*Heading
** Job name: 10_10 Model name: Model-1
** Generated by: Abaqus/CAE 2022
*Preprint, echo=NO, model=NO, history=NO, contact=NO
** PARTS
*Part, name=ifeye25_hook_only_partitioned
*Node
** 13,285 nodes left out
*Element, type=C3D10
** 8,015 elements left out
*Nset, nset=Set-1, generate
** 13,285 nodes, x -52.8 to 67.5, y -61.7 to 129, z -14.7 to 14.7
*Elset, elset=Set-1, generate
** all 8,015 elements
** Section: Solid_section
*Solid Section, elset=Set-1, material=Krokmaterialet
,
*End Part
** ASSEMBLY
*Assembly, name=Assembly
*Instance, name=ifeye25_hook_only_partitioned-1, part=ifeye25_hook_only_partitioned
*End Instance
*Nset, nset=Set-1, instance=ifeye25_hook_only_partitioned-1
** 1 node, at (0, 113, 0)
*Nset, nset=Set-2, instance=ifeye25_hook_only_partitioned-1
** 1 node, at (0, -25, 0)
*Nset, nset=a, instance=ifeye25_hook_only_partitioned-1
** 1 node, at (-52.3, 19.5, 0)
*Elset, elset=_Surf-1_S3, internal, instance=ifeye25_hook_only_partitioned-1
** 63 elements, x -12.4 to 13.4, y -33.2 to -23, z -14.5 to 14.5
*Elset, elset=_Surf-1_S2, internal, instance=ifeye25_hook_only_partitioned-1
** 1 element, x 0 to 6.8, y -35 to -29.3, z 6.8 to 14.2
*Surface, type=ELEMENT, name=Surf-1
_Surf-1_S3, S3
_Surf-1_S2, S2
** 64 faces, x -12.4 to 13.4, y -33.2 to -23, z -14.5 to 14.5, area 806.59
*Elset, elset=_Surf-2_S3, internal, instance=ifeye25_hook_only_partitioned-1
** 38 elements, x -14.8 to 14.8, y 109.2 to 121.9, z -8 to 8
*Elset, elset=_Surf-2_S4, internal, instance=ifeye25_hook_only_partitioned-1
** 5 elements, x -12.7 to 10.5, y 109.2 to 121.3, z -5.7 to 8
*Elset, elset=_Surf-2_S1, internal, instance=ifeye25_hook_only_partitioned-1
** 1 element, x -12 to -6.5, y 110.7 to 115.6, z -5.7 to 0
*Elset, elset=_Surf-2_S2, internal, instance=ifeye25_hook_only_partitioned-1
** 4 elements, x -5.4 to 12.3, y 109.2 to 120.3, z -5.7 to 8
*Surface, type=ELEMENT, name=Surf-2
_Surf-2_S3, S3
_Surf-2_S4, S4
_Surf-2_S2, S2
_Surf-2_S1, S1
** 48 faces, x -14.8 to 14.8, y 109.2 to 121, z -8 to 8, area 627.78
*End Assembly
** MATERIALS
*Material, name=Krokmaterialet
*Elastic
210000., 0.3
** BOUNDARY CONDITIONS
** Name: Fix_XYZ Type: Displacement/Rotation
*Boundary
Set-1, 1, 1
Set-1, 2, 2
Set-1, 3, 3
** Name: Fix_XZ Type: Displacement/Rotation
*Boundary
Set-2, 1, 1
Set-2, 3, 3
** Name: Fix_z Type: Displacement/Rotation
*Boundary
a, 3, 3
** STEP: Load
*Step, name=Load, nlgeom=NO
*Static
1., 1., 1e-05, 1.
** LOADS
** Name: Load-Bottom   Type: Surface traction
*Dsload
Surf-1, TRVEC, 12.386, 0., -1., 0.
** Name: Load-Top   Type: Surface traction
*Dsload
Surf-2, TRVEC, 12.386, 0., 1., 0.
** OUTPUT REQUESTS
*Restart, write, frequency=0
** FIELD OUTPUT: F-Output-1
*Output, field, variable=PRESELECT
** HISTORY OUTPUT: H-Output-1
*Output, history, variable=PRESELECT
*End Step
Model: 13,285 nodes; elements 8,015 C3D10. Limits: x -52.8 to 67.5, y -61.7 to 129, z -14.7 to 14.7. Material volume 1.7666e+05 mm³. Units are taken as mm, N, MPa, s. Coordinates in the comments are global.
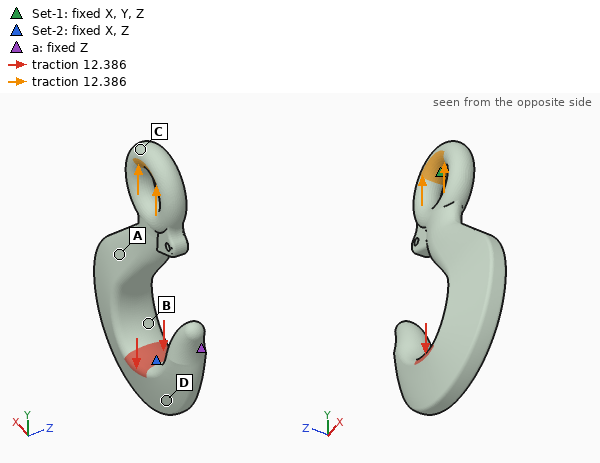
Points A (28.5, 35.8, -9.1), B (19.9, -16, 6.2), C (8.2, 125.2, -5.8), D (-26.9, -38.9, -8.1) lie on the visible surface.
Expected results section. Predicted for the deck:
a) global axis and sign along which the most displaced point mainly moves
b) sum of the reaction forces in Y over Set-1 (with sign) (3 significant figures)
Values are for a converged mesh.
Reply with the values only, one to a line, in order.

-Y
2210 N
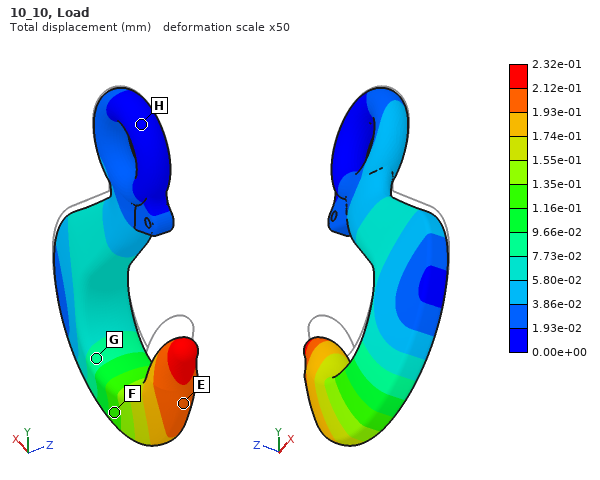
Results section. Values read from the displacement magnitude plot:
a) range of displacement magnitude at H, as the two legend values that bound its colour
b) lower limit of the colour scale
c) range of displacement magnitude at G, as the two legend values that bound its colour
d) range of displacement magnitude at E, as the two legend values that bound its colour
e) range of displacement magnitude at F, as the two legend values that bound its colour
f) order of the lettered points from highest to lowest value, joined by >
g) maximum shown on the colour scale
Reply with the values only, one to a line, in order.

0.00e+00 to 1.93e-02 mm
0.00e+00 mm
7.73e-02 to 9.66e-02 mm
1.93e-01 to 2.12e-01 mm
1.16e-01 to 1.35e-01 mm
E > F > G > H
2.32e-01 mm
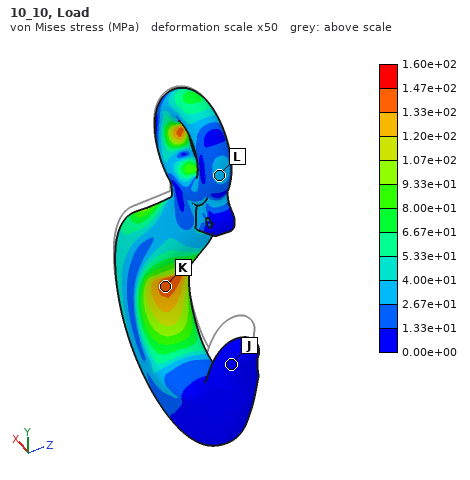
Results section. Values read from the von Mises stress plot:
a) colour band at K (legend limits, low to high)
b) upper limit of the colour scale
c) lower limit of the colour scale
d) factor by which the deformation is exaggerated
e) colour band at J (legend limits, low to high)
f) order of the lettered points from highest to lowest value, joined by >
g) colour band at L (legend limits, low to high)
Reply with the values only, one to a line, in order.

1.33e+02 to 1.47e+02 MPa
1.60e+02 MPa
0.00e+00 MPa
50
0.00e+00 to 1.33e+01 MPa
K > L > J
2.67e+01 to 4.00e+01 MPa
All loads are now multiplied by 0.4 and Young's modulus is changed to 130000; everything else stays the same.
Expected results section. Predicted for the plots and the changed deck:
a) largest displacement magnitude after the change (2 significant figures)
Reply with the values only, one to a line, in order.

0.15 mm
